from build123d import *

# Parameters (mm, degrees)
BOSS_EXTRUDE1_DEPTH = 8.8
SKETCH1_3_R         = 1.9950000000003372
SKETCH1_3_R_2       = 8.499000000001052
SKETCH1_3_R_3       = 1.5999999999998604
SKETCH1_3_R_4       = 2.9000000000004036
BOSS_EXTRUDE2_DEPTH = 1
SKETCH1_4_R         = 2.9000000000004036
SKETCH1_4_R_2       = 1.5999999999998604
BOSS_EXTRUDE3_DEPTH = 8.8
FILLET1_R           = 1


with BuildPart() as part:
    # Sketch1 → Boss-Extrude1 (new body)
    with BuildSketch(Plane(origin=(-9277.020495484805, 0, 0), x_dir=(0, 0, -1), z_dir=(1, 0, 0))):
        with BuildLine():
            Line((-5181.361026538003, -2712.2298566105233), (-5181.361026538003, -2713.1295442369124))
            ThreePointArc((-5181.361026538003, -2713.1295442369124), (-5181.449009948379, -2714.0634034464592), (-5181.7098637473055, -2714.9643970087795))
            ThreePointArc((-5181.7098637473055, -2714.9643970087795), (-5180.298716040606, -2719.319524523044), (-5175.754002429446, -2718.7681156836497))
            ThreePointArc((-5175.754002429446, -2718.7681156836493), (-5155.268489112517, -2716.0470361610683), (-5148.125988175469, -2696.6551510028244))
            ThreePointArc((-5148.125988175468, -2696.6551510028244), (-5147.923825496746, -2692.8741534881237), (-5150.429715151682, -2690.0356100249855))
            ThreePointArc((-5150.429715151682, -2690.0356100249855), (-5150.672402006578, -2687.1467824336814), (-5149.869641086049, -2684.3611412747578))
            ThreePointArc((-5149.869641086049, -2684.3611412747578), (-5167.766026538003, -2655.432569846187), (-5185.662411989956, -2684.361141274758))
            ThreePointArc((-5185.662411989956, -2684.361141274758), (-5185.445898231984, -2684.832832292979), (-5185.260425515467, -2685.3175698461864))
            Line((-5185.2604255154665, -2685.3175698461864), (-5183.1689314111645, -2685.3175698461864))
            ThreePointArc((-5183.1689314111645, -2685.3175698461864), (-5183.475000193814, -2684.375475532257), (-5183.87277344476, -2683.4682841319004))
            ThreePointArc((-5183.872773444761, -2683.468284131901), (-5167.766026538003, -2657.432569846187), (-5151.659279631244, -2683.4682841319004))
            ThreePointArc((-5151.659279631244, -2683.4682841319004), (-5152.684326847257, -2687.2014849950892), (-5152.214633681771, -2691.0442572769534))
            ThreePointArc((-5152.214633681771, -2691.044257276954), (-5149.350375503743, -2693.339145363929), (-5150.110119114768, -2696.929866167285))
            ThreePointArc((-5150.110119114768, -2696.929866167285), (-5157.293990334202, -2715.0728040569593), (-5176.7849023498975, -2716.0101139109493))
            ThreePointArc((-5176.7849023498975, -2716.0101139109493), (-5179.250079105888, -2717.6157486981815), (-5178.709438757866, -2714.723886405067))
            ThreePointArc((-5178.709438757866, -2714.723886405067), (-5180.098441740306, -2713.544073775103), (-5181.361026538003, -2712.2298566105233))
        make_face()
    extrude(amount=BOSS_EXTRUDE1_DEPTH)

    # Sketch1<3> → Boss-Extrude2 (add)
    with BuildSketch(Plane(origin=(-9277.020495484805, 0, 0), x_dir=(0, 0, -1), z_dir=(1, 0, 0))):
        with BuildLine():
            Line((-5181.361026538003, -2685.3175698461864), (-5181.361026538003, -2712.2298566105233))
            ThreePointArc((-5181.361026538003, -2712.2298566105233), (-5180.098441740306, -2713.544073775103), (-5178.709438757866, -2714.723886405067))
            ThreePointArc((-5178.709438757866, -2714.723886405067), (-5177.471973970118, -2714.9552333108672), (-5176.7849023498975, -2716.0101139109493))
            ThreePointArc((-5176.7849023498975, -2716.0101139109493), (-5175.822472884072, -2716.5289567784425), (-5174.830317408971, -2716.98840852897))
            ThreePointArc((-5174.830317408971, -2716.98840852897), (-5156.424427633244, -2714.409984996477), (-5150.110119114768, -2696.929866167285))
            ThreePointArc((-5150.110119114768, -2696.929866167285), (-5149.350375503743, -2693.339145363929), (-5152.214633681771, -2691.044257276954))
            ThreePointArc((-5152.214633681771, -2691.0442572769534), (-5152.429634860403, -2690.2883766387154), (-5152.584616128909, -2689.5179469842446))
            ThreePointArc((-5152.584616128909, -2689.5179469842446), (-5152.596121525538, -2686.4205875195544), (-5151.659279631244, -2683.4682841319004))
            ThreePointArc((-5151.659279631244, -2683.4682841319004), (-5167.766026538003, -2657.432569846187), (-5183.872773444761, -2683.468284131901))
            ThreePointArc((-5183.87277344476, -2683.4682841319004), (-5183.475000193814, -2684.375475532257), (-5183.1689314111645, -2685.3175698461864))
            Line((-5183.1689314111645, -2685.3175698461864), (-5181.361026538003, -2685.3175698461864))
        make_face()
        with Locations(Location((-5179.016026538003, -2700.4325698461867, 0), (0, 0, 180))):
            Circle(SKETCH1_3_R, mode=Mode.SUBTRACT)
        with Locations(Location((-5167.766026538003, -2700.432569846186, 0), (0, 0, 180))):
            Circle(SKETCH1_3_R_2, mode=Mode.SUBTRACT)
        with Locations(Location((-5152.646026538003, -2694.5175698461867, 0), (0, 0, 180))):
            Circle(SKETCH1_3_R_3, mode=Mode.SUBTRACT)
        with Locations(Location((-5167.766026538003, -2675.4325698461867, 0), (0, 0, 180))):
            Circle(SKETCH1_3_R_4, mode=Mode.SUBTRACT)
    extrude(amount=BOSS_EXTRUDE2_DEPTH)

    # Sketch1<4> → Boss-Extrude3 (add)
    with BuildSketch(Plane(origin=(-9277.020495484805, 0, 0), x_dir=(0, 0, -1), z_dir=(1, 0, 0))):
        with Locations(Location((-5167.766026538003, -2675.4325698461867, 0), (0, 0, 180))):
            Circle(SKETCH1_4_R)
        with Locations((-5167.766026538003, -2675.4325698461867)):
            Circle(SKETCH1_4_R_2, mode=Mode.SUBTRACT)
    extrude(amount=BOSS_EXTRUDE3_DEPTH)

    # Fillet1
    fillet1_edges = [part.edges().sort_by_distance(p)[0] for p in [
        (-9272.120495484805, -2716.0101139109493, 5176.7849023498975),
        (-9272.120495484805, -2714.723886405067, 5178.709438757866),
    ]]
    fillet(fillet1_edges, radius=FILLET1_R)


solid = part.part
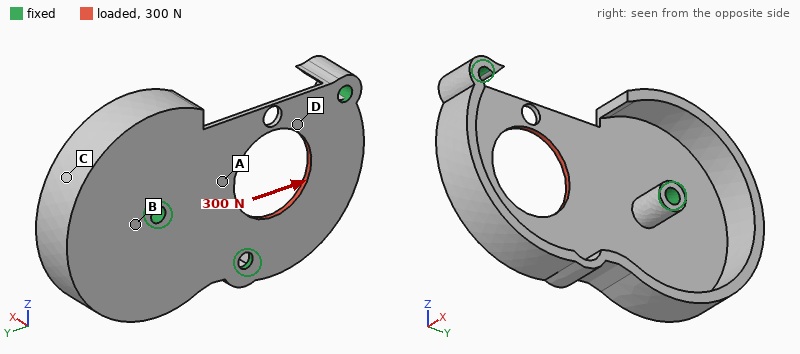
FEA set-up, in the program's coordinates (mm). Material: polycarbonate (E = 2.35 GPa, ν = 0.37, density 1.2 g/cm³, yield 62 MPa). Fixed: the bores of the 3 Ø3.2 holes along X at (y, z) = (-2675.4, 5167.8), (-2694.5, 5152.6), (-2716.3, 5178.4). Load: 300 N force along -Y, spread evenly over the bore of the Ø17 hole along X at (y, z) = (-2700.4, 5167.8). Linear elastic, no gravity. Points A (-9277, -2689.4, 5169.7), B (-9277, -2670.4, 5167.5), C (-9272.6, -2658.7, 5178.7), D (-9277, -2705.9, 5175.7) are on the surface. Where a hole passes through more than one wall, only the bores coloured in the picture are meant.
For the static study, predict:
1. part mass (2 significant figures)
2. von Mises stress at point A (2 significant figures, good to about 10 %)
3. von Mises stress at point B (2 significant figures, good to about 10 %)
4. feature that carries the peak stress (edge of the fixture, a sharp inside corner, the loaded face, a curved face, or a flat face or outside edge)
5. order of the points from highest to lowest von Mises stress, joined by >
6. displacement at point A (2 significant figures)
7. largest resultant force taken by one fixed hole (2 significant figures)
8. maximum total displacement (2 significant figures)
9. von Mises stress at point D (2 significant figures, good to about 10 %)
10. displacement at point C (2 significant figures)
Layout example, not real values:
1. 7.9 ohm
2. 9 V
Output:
1. 5.0 g
2. 6.7 MPa
3. 3.1 MPa
4. a curved face
5. D > A > B > C
6. 0.046 mm
7. 110 N
8. 0.10 mm
9. 8.4 MPa
10. 0.038 mm
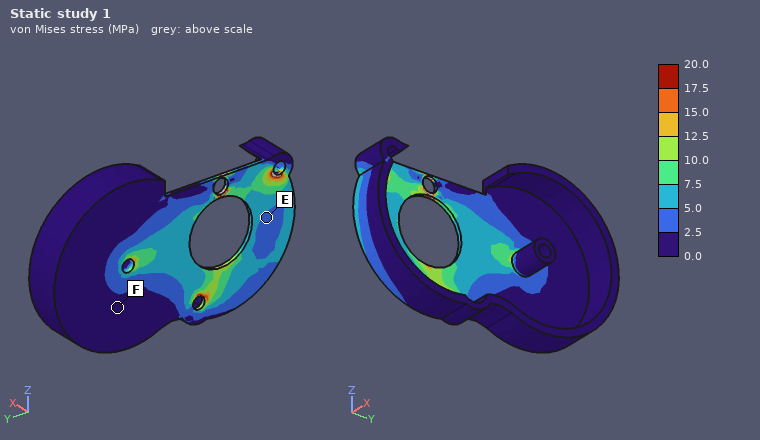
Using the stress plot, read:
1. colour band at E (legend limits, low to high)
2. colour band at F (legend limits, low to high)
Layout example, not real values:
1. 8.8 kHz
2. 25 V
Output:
1. 2.5 to 5.0 MPa
2. 0.0 to 2.5 MPa
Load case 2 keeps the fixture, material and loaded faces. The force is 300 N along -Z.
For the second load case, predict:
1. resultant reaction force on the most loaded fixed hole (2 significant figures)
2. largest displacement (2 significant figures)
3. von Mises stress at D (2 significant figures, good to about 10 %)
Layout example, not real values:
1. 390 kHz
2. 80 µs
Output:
1. 130 N
2. 0.26 mm
3. 11 MPa
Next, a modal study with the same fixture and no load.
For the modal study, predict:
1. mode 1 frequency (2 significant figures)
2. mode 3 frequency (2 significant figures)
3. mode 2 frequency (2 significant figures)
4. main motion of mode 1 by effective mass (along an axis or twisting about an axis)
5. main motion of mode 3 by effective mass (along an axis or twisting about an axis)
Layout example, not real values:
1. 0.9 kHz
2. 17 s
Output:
1. 490 Hz
2. 990 Hz
3. 560 Hz
4. along X
5. along X
